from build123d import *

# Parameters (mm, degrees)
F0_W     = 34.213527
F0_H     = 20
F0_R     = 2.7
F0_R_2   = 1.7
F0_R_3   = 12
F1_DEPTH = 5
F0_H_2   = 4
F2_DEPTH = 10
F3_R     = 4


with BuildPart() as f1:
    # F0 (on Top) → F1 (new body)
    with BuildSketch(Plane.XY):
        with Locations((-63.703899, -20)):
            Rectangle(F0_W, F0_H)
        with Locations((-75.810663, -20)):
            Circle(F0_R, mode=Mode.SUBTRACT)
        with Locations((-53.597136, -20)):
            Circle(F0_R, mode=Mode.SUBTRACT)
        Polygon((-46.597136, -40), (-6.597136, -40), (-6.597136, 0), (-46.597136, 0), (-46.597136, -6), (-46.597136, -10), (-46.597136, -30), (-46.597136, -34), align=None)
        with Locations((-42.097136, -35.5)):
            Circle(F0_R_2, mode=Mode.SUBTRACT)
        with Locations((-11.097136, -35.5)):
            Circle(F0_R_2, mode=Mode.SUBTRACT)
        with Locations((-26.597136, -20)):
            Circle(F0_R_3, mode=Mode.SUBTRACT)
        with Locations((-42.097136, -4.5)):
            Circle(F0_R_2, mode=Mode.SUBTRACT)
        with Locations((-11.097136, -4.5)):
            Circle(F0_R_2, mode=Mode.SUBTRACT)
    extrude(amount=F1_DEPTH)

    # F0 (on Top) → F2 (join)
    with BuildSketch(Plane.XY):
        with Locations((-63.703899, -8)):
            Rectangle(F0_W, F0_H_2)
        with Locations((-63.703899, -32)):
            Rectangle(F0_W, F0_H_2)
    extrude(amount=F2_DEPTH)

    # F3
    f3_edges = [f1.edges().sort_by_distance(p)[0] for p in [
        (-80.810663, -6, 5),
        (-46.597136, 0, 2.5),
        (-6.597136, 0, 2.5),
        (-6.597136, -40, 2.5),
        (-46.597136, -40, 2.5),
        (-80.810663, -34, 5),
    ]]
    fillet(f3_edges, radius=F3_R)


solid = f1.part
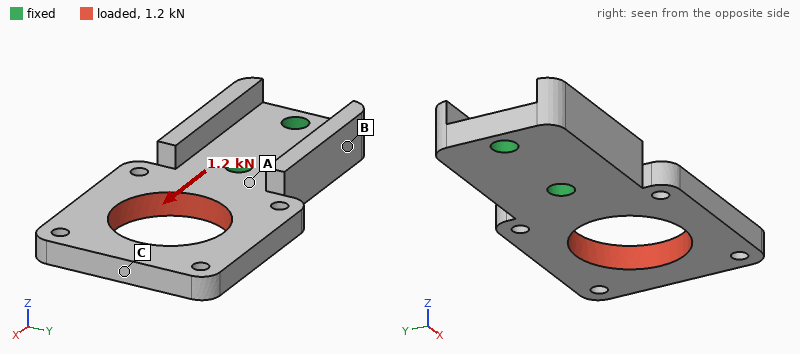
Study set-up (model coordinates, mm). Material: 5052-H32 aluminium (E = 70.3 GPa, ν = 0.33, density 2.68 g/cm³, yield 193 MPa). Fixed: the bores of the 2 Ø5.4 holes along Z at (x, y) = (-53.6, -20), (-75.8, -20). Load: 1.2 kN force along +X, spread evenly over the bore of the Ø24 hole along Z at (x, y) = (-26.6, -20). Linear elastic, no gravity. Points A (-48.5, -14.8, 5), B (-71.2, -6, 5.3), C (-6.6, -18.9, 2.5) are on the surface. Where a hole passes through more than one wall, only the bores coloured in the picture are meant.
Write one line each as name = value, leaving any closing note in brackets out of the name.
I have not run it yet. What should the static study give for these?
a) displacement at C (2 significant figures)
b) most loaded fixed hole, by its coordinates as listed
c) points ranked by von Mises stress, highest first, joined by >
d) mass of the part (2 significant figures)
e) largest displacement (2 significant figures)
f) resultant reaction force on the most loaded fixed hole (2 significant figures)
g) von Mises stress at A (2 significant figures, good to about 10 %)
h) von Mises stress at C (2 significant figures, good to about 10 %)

displacement at C = 14 µm
most loaded fixed hole, by its coordinates as listed = (-53.6, -20)
points ranked by von Mises stress, highest first, joined by > = C > A > B
mass of the part = 30 g
largest displacement = 15 µm
resultant reaction force on the most loaded fixed hole = 900 N
von Mises stress at A = 7.9 MPa
von Mises stress at C = 18 MPa
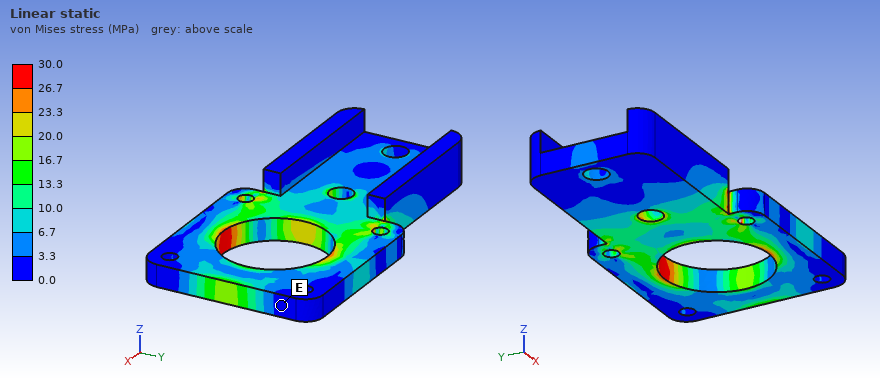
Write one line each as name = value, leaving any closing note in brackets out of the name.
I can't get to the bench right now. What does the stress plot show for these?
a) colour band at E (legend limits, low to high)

colour band at E = 0.0 to 3.3 MPa
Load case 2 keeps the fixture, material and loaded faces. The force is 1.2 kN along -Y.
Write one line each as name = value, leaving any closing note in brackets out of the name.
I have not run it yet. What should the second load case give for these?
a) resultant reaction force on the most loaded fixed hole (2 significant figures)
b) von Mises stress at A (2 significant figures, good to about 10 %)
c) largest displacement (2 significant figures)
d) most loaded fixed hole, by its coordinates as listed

resultant reaction force on the most loaded fixed hole = 2.2 kN
von Mises stress at A = 29 MPa
largest displacement = 0.10 mm
most loaded fixed hole, by its coordinates as listed = (-53.6, -20)
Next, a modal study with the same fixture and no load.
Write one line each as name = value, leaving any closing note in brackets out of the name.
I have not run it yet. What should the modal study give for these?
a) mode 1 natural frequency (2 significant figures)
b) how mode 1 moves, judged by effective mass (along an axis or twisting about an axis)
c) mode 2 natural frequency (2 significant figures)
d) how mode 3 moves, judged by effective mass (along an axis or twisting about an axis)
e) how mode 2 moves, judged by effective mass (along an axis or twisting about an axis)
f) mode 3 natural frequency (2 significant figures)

mode 1 natural frequency = 1700 Hz
how mode 1 moves, judged by effective mass = along Z
mode 2 natural frequency = 3500 Hz
how mode 3 moves, judged by effective mass = along Y
how mode 2 moves, judged by effective mass = twisting about X
mode 3 natural frequency = 5100 Hz
